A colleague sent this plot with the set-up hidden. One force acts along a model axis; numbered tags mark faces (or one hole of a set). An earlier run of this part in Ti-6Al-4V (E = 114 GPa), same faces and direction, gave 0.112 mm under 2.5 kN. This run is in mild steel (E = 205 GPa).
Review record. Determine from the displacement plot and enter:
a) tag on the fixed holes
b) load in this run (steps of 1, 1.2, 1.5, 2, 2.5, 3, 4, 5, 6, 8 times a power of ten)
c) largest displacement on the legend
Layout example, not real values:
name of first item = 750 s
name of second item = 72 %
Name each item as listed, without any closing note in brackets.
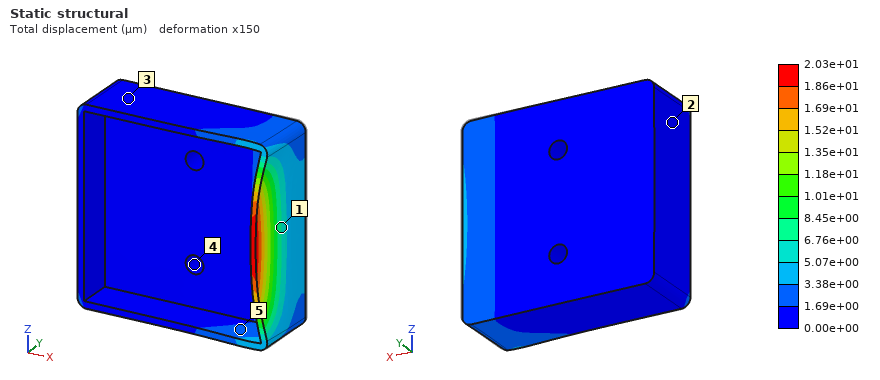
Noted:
tag on the fixed holes = 4
load in this run = 800 N
largest displacement on the legend = 2.03e+01 µm
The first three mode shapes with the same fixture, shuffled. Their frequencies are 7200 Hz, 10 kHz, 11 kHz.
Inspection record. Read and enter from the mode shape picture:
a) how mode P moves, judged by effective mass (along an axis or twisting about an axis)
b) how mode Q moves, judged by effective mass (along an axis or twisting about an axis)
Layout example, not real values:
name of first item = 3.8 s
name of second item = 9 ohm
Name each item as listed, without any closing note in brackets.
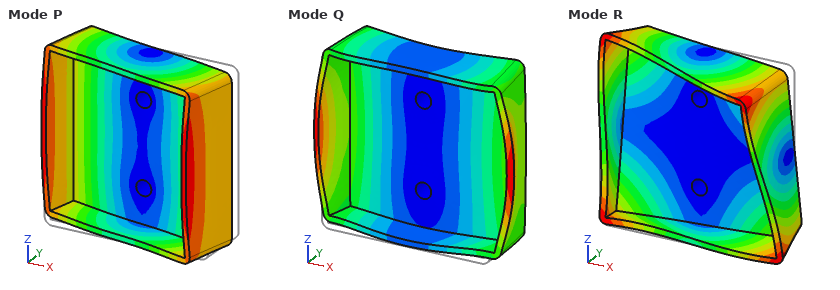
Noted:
how mode P moves, judged by effective mass = twisting about Z
how mode Q moves, judged by effective mass = along Y
